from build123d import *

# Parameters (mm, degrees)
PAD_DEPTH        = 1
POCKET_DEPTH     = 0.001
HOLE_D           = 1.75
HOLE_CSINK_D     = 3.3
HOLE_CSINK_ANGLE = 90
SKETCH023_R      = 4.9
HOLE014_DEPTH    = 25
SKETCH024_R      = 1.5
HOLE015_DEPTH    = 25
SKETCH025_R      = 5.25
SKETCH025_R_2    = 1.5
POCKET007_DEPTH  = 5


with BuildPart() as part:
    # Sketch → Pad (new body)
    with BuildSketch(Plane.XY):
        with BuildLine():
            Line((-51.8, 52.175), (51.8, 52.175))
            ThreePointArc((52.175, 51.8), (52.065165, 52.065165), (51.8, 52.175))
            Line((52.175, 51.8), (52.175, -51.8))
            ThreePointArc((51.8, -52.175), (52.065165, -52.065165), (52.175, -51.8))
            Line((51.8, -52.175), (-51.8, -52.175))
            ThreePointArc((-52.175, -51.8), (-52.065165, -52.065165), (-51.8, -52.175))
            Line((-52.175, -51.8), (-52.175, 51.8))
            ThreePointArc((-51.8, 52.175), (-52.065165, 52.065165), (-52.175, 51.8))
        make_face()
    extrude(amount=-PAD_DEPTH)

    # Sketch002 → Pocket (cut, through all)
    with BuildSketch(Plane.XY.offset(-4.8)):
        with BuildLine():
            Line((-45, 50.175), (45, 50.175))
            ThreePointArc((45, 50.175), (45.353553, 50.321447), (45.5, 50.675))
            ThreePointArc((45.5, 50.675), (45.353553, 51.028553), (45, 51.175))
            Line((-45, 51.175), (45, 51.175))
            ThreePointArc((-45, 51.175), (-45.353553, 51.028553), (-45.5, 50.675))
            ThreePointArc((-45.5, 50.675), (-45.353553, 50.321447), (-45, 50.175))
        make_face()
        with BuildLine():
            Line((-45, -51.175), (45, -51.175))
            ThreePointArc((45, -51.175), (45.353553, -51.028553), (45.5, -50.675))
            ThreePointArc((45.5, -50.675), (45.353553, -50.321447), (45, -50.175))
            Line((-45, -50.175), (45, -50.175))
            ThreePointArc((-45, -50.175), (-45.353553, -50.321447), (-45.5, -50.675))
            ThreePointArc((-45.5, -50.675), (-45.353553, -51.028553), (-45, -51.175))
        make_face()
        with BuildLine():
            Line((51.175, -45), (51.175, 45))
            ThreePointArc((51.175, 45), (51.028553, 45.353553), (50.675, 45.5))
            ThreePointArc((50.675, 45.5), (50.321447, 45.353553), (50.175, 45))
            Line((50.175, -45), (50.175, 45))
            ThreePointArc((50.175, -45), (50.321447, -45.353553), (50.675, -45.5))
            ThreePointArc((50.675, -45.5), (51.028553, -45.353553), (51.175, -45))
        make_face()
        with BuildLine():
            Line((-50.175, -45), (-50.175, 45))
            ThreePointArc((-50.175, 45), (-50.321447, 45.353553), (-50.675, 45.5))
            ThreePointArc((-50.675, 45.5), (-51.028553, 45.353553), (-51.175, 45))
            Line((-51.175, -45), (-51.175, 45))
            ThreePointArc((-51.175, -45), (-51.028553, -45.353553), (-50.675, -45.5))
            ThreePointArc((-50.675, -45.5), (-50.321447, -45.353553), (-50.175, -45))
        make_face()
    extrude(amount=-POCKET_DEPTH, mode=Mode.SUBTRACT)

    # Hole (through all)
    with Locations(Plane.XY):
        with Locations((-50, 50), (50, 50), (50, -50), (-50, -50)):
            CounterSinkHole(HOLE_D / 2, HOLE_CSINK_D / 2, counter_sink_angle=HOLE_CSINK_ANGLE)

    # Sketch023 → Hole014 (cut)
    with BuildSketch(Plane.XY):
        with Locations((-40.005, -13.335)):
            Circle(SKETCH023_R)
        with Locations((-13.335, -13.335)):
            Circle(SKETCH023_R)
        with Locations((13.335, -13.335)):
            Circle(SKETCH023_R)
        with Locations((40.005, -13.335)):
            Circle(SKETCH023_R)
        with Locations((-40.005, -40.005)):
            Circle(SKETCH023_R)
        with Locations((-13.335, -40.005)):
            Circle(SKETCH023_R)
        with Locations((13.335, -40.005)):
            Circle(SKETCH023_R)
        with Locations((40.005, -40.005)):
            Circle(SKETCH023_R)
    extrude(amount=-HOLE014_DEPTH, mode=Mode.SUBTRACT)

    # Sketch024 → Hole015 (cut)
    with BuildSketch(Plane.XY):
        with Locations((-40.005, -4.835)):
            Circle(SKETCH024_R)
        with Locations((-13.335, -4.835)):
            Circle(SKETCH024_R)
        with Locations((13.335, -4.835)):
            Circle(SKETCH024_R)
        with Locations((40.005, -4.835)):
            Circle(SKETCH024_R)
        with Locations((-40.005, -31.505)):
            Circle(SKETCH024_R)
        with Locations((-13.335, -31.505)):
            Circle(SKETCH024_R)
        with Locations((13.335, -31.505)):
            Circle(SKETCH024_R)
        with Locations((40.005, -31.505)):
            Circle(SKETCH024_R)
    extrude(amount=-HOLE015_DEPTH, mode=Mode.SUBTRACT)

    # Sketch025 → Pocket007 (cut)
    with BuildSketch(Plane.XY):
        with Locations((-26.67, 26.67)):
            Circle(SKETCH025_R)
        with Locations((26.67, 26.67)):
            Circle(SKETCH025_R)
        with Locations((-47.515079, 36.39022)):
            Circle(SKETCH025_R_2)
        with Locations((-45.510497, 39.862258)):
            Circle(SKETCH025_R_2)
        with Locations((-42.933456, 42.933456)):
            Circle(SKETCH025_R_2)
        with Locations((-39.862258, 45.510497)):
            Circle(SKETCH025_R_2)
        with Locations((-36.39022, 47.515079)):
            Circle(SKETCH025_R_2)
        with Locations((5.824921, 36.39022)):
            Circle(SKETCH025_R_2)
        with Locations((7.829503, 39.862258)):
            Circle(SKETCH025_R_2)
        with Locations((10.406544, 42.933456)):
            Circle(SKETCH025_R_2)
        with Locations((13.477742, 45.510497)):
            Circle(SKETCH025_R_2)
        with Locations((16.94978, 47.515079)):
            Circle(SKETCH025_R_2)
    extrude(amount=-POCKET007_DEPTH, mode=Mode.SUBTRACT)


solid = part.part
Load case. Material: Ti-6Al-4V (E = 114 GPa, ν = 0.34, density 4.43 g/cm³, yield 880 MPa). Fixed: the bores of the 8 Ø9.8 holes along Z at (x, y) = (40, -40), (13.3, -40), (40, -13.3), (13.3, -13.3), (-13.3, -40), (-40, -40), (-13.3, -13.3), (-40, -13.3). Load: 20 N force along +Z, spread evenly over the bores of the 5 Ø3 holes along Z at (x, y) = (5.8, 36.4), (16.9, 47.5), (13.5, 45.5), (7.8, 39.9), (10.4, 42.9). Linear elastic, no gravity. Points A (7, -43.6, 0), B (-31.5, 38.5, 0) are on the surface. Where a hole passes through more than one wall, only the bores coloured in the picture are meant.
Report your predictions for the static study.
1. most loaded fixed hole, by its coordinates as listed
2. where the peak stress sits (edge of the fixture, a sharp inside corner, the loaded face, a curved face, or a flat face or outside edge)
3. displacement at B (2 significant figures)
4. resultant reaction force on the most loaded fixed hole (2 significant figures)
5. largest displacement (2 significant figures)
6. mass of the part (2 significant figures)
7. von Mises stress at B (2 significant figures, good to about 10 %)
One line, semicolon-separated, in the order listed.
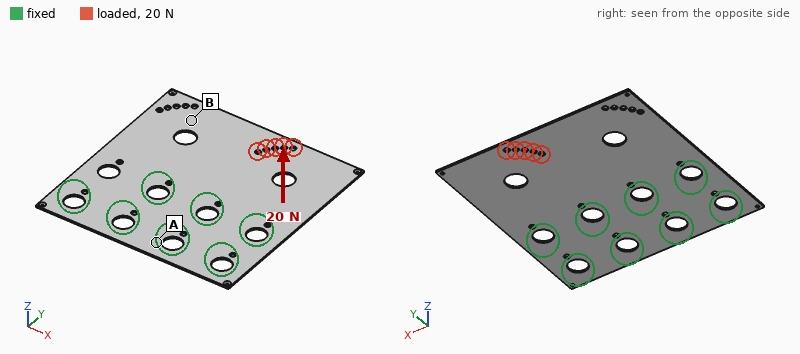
(13.3, -13.3); a curved face; 0.68 mm; 10 N; 1.5 mm; 44 g; 17 MPa
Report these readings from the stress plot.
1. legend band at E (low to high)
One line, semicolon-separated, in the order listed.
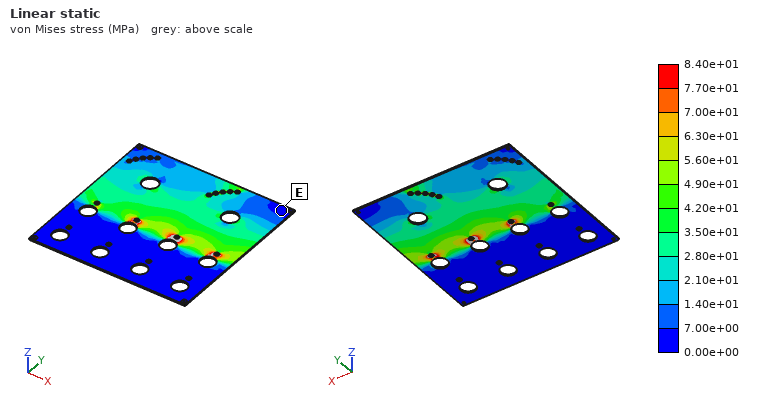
0.00e+00 to 7.00e+00 MPa
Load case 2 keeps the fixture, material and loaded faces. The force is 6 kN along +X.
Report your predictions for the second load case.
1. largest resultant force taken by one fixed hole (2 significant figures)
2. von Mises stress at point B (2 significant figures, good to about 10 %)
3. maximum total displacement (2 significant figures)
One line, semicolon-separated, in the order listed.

3.7 kN; 74 MPa; 0.16 mm
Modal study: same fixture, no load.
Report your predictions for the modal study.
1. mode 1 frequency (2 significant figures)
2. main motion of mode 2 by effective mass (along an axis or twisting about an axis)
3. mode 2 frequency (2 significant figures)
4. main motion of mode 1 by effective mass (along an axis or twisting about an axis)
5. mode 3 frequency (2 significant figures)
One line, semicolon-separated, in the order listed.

220 Hz; twisting about Y; 370 Hz; along Z; 770 Hz
